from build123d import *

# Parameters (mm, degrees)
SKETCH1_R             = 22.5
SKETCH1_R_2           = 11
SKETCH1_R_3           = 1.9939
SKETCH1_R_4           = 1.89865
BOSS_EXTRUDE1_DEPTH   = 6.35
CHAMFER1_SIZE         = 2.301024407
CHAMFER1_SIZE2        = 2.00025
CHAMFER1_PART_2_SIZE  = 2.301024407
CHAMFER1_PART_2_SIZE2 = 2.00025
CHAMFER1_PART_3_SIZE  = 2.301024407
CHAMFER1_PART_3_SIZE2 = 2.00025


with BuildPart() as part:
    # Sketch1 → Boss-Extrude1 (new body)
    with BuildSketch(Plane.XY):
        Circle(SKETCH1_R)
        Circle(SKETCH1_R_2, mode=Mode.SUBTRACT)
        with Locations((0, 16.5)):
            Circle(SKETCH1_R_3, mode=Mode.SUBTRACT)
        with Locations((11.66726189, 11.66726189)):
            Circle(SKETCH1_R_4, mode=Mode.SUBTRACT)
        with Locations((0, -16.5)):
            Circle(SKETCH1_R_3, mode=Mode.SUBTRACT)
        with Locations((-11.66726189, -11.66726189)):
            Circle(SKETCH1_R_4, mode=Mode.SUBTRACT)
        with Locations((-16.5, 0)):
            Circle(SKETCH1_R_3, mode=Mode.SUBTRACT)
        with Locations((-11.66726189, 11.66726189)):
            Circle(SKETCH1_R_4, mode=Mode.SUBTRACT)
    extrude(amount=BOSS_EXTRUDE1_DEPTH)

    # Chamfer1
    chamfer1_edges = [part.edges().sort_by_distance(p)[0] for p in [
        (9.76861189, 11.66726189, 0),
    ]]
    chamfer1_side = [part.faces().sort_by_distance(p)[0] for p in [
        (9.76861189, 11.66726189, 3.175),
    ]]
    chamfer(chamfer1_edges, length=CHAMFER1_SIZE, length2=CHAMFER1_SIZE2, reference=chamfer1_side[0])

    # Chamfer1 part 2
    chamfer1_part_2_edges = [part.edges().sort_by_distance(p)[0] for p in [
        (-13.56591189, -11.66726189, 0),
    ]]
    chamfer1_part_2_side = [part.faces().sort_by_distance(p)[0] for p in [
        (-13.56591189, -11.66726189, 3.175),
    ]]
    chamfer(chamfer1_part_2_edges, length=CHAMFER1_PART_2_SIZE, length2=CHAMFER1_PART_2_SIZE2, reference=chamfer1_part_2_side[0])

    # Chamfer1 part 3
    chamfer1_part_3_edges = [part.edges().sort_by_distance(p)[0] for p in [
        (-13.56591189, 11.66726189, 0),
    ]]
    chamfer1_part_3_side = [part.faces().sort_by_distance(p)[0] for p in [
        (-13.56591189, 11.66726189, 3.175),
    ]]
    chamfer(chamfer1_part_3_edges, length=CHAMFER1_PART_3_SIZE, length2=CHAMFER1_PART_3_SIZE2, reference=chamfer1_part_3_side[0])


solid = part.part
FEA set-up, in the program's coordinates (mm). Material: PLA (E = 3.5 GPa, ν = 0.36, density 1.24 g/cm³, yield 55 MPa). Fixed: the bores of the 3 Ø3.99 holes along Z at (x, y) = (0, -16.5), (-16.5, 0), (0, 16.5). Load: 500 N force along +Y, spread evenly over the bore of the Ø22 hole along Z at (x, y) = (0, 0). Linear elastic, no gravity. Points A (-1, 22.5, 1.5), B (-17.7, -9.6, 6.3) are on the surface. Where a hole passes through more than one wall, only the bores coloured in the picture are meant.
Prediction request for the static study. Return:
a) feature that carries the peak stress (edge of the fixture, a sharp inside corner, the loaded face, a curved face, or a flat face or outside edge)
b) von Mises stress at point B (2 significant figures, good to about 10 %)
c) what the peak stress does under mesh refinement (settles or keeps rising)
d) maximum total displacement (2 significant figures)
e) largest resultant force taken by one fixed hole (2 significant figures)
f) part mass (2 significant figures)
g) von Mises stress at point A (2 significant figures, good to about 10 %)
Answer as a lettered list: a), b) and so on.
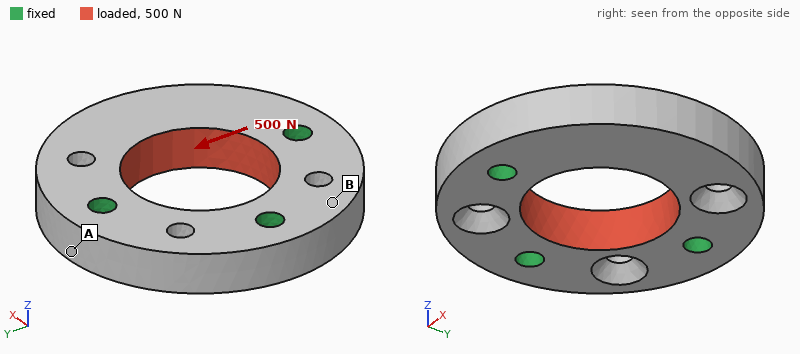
a) edge of the fixture
b) 0.69 MPa
c) keeps rising
d) 24 µm
e) 200 N
f) 8.8 g
g) 2.1 MPa
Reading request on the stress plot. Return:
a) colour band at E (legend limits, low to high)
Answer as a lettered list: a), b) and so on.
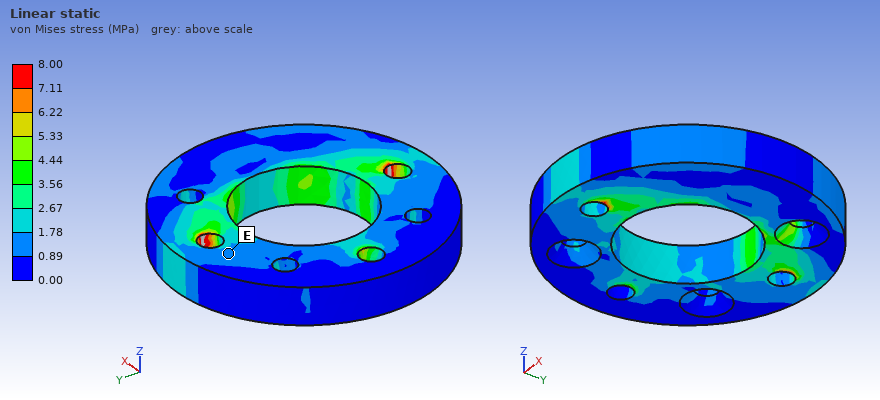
a) 0.89 to 1.78 MPa
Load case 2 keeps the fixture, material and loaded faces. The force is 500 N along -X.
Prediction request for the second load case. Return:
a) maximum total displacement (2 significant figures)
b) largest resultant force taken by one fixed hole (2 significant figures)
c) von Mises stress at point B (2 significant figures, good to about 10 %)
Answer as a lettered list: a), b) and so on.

a) 17 µm
b) 190 N
c) 0.76 MPa
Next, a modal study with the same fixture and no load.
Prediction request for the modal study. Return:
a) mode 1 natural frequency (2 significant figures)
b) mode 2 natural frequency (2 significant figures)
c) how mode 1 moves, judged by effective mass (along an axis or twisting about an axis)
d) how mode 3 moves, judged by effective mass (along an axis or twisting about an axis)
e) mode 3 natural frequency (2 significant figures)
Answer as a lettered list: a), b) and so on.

a) 3000 Hz
b) 7300 Hz
c) along Z
d) along Y
e) 8000 Hz
